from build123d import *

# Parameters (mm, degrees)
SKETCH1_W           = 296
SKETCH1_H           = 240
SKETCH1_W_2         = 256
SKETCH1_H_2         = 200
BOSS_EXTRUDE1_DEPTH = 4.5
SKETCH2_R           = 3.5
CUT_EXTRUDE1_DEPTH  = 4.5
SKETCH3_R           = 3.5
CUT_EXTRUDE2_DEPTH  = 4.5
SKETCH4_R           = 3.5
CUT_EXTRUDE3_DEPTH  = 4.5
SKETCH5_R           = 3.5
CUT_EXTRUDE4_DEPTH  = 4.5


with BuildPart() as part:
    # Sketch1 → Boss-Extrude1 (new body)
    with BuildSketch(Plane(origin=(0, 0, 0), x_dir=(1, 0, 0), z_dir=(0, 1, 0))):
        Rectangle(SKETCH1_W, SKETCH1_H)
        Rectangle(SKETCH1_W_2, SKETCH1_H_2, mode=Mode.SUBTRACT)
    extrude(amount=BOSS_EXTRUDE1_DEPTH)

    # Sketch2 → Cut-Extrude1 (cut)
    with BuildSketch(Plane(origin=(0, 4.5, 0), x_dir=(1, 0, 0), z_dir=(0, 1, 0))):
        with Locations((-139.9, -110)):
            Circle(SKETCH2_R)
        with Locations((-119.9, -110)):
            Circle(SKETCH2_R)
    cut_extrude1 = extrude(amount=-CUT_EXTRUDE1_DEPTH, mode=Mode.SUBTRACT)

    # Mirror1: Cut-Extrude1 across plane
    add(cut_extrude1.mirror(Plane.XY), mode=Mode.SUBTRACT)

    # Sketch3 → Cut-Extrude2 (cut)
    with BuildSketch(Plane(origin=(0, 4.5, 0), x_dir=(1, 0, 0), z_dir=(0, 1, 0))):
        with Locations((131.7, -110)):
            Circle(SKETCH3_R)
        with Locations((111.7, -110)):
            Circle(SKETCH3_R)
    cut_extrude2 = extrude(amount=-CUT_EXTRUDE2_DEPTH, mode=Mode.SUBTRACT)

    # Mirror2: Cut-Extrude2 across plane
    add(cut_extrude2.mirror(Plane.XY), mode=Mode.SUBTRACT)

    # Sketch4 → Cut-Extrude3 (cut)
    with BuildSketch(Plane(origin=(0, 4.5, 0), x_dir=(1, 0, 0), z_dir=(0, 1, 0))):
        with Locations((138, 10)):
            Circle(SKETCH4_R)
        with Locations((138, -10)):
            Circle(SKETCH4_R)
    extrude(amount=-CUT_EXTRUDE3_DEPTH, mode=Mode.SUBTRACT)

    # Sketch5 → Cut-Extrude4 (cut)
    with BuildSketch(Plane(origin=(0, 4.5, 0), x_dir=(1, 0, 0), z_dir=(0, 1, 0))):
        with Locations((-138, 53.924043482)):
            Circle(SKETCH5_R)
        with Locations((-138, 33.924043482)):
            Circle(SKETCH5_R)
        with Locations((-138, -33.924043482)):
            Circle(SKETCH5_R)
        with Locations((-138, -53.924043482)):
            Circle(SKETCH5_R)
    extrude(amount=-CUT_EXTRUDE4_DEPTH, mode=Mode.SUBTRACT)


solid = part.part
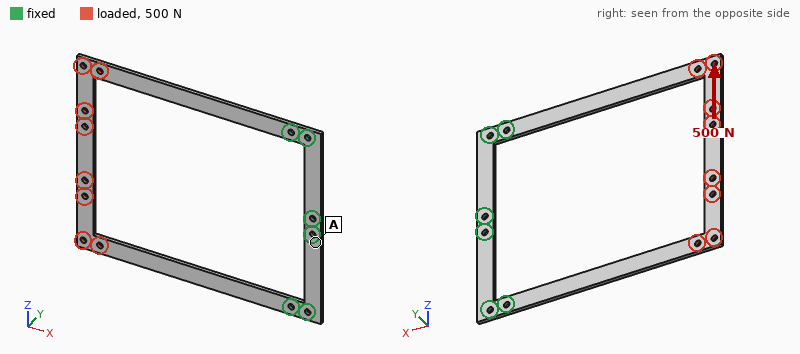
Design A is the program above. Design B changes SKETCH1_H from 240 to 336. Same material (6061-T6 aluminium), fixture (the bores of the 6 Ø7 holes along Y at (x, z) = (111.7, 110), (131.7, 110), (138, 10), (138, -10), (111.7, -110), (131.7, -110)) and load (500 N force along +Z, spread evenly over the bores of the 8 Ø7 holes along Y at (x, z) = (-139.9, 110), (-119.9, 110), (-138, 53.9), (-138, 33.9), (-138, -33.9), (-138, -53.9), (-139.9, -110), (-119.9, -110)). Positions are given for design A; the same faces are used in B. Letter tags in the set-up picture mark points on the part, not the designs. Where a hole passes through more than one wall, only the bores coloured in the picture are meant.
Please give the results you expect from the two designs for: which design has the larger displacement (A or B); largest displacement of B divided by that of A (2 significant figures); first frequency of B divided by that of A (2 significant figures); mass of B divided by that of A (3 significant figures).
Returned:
A
0.13
1.2
2.47
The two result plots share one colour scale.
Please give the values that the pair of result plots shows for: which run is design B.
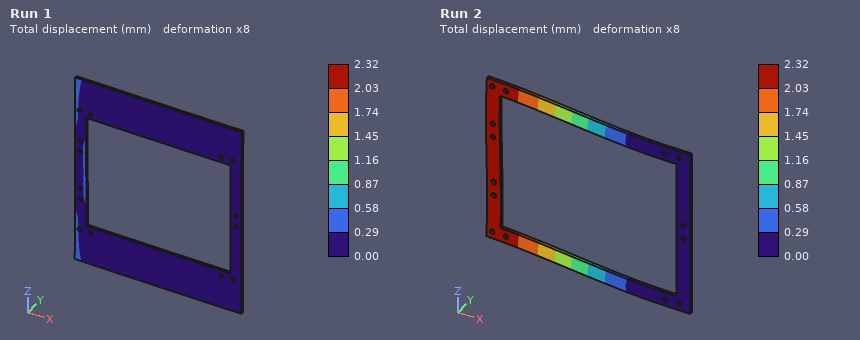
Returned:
Run 1
